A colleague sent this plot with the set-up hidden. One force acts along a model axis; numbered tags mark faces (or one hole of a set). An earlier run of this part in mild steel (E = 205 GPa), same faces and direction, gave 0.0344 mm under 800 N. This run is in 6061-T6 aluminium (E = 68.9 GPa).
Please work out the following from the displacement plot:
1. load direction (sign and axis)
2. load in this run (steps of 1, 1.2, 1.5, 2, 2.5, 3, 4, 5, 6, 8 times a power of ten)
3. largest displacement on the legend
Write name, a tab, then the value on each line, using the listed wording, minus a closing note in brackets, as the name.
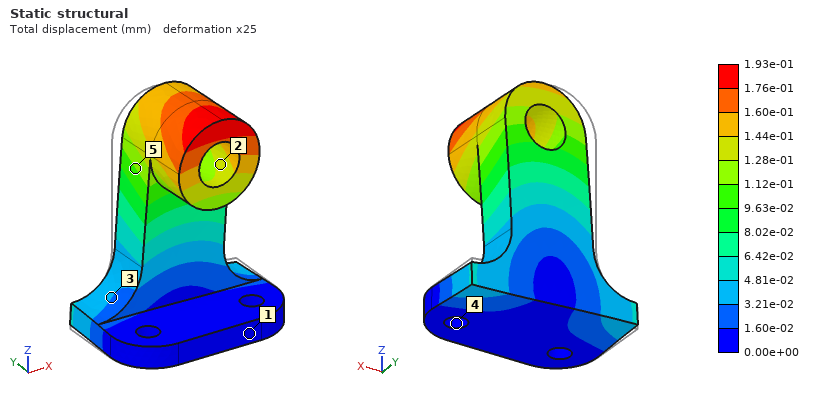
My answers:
load direction	+X
load in this run	1.5 kN
largest displacement on the legend	1.93e-01 mm
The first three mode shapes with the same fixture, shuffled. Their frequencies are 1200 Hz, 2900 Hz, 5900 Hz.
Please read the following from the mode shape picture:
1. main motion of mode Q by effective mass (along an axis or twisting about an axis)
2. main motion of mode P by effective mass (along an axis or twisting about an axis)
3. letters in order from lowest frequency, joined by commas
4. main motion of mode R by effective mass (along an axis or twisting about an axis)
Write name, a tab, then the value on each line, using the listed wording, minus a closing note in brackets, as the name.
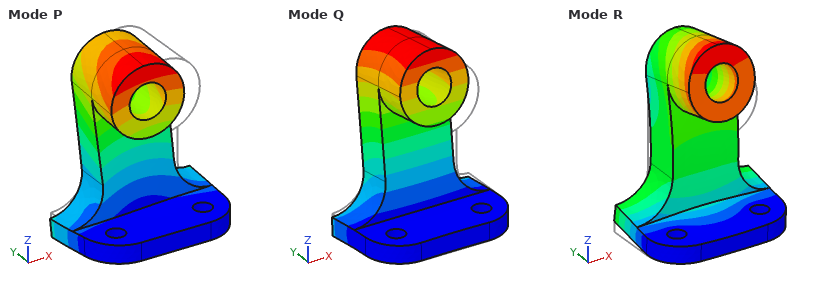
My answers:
main motion of mode Q by effective mass	along Y
main motion of mode P by effective mass	along X
letters in order from lowest frequency, joined by commas	Q, P, R
main motion of mode R by effective mass	along Z
